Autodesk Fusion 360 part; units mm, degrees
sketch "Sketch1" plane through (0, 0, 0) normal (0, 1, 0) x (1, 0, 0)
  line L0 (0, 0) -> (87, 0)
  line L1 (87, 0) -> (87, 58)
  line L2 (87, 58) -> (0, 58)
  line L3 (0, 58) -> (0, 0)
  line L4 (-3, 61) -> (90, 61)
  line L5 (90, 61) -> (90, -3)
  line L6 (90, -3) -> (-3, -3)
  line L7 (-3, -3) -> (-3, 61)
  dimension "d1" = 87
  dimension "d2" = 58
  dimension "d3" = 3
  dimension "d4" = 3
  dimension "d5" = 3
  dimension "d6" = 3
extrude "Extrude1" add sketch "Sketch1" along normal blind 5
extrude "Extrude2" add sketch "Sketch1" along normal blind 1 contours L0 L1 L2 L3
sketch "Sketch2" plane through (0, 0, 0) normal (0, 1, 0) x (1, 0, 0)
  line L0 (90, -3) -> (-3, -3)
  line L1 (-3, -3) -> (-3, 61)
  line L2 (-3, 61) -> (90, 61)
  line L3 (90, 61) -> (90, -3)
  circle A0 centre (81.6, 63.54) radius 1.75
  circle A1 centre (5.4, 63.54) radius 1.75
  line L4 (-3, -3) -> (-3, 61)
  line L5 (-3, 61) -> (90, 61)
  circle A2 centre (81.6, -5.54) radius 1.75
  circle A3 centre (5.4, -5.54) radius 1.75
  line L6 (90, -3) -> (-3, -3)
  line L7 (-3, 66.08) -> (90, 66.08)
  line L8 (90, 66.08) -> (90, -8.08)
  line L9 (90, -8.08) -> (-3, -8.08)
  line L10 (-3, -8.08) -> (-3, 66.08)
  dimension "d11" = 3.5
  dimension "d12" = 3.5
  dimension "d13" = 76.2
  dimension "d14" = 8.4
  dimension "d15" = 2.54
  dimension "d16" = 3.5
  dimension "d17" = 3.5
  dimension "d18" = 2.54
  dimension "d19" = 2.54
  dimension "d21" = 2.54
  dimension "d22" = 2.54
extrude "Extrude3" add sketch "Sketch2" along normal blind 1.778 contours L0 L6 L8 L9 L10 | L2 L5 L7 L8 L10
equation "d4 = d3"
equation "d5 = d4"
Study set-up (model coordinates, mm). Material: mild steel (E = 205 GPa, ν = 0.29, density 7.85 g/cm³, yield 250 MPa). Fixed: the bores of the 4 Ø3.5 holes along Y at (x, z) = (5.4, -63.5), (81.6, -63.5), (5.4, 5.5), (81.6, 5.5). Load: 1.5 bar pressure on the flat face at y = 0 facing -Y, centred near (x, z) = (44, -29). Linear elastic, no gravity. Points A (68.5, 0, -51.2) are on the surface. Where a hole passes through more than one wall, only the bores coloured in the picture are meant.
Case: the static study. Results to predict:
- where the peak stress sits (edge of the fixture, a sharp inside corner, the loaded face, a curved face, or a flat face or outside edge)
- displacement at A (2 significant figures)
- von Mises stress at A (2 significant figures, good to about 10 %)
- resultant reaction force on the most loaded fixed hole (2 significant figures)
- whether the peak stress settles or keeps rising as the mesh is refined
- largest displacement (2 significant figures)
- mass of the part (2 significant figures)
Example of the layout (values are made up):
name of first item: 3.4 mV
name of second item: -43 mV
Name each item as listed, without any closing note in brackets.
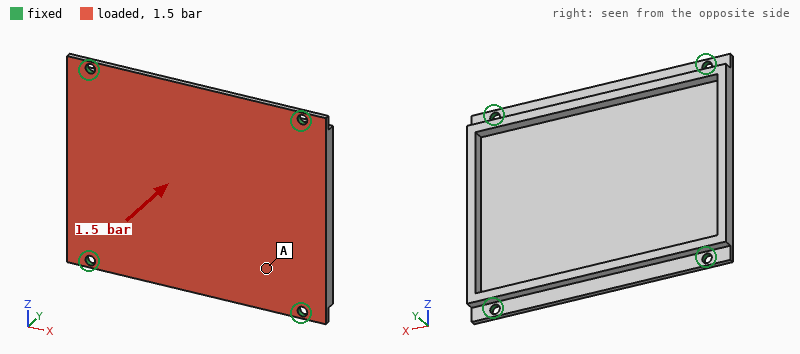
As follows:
where the peak stress sits: edge of the fixture
displacement at A: 0.10 mm
von Mises stress at A: 42 MPa
resultant reaction force on the most loaded fixed hole: 270 N
whether the peak stress settles or keeps rising as the mesh is refined: keeps rising
largest displacement: 0.40 mm
mass of the part: 88 g
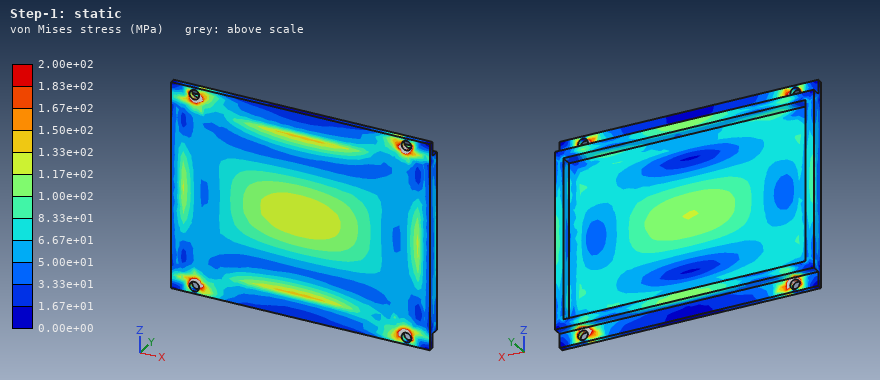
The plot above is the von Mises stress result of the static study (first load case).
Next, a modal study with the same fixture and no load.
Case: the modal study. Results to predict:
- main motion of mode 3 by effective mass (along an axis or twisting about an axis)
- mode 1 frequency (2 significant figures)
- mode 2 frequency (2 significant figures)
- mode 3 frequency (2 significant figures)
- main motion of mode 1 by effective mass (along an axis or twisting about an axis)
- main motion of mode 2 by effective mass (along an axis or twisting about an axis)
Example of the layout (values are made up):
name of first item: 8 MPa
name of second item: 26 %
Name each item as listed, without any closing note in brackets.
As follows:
main motion of mode 3 by effective mass: twisting about X
mode 1 frequency: 1400 Hz
mode 2 frequency: 2500 Hz
mode 3 frequency: 2700 Hz
main motion of mode 1 by effective mass: along Y
main motion of mode 2 by effective mass: twisting about Z
